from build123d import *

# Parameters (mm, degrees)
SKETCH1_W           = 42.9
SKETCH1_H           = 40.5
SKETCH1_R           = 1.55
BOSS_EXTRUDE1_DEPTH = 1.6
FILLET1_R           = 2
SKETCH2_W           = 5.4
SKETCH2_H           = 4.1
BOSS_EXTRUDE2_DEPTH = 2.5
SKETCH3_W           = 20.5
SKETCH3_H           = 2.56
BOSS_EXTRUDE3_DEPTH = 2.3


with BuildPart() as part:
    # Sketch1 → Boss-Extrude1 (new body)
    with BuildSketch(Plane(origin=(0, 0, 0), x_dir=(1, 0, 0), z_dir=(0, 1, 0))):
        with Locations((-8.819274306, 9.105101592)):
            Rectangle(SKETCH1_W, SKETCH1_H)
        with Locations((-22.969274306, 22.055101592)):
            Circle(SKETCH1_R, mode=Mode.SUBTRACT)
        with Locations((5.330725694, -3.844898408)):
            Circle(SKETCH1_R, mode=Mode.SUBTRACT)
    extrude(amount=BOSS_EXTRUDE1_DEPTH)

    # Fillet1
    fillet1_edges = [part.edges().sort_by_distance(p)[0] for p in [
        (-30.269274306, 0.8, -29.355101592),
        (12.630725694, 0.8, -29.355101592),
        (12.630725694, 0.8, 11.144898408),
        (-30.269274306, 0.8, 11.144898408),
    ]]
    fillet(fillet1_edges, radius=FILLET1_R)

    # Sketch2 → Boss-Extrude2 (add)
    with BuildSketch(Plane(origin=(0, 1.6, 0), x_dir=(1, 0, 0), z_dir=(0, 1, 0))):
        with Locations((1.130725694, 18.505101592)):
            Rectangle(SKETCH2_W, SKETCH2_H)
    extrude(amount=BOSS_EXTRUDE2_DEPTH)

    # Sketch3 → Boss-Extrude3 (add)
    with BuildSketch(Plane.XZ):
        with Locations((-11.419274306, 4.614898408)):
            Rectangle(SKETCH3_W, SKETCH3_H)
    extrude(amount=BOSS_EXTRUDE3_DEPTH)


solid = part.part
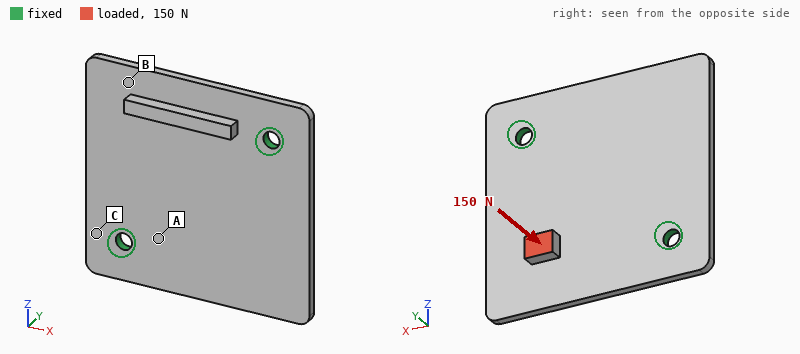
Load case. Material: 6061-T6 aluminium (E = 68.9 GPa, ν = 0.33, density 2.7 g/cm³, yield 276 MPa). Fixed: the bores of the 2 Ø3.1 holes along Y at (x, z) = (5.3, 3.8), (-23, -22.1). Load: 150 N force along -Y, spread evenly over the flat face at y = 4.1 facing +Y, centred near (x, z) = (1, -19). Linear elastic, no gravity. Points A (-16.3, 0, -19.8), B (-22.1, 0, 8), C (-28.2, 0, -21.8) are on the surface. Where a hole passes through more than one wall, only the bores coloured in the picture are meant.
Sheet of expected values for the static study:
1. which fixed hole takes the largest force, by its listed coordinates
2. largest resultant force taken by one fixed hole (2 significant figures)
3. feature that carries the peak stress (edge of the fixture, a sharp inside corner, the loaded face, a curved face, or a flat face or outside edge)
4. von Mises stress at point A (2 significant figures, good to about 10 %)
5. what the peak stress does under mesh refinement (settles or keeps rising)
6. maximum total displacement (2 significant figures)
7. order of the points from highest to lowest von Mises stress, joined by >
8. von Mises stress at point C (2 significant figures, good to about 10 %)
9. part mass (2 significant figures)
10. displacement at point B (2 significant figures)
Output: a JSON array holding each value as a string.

["(5.3, 3.8)", "80 N", "edge of the fixture", "83 MPa", "keeps rising", "0.62 mm", "A > C > B", "36 MPa", "7.9 g", "0.12 mm"]
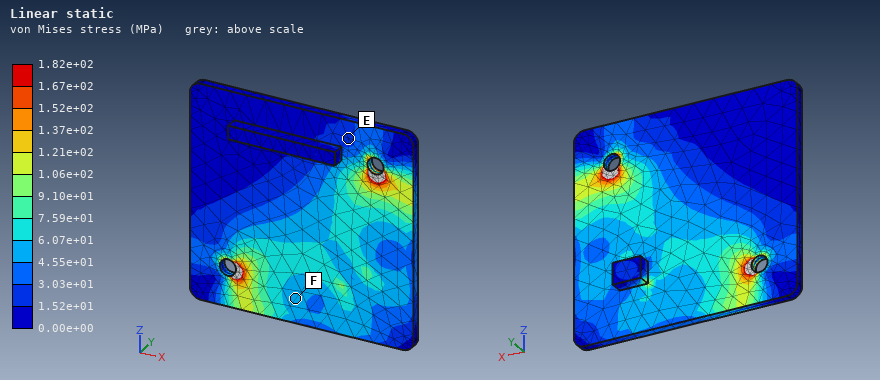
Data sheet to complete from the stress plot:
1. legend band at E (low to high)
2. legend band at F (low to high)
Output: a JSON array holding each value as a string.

["1.52e+01 to 3.03e+01 MPa", "4.55e+01 to 6.07e+01 MPa"]
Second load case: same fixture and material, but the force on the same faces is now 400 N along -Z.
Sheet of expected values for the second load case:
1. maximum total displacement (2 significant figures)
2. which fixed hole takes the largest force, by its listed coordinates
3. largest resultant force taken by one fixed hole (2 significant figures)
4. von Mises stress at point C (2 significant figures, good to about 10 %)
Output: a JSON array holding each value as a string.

["0.40 mm", "(5.3, 3.8)", "300 N", "20 MPa"]
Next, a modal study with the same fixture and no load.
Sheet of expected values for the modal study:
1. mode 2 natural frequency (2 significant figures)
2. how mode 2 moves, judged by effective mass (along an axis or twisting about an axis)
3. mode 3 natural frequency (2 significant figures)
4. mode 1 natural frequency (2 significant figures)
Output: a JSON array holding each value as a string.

["2500 Hz", "along Y", "7100 Hz", "1900 Hz"]
